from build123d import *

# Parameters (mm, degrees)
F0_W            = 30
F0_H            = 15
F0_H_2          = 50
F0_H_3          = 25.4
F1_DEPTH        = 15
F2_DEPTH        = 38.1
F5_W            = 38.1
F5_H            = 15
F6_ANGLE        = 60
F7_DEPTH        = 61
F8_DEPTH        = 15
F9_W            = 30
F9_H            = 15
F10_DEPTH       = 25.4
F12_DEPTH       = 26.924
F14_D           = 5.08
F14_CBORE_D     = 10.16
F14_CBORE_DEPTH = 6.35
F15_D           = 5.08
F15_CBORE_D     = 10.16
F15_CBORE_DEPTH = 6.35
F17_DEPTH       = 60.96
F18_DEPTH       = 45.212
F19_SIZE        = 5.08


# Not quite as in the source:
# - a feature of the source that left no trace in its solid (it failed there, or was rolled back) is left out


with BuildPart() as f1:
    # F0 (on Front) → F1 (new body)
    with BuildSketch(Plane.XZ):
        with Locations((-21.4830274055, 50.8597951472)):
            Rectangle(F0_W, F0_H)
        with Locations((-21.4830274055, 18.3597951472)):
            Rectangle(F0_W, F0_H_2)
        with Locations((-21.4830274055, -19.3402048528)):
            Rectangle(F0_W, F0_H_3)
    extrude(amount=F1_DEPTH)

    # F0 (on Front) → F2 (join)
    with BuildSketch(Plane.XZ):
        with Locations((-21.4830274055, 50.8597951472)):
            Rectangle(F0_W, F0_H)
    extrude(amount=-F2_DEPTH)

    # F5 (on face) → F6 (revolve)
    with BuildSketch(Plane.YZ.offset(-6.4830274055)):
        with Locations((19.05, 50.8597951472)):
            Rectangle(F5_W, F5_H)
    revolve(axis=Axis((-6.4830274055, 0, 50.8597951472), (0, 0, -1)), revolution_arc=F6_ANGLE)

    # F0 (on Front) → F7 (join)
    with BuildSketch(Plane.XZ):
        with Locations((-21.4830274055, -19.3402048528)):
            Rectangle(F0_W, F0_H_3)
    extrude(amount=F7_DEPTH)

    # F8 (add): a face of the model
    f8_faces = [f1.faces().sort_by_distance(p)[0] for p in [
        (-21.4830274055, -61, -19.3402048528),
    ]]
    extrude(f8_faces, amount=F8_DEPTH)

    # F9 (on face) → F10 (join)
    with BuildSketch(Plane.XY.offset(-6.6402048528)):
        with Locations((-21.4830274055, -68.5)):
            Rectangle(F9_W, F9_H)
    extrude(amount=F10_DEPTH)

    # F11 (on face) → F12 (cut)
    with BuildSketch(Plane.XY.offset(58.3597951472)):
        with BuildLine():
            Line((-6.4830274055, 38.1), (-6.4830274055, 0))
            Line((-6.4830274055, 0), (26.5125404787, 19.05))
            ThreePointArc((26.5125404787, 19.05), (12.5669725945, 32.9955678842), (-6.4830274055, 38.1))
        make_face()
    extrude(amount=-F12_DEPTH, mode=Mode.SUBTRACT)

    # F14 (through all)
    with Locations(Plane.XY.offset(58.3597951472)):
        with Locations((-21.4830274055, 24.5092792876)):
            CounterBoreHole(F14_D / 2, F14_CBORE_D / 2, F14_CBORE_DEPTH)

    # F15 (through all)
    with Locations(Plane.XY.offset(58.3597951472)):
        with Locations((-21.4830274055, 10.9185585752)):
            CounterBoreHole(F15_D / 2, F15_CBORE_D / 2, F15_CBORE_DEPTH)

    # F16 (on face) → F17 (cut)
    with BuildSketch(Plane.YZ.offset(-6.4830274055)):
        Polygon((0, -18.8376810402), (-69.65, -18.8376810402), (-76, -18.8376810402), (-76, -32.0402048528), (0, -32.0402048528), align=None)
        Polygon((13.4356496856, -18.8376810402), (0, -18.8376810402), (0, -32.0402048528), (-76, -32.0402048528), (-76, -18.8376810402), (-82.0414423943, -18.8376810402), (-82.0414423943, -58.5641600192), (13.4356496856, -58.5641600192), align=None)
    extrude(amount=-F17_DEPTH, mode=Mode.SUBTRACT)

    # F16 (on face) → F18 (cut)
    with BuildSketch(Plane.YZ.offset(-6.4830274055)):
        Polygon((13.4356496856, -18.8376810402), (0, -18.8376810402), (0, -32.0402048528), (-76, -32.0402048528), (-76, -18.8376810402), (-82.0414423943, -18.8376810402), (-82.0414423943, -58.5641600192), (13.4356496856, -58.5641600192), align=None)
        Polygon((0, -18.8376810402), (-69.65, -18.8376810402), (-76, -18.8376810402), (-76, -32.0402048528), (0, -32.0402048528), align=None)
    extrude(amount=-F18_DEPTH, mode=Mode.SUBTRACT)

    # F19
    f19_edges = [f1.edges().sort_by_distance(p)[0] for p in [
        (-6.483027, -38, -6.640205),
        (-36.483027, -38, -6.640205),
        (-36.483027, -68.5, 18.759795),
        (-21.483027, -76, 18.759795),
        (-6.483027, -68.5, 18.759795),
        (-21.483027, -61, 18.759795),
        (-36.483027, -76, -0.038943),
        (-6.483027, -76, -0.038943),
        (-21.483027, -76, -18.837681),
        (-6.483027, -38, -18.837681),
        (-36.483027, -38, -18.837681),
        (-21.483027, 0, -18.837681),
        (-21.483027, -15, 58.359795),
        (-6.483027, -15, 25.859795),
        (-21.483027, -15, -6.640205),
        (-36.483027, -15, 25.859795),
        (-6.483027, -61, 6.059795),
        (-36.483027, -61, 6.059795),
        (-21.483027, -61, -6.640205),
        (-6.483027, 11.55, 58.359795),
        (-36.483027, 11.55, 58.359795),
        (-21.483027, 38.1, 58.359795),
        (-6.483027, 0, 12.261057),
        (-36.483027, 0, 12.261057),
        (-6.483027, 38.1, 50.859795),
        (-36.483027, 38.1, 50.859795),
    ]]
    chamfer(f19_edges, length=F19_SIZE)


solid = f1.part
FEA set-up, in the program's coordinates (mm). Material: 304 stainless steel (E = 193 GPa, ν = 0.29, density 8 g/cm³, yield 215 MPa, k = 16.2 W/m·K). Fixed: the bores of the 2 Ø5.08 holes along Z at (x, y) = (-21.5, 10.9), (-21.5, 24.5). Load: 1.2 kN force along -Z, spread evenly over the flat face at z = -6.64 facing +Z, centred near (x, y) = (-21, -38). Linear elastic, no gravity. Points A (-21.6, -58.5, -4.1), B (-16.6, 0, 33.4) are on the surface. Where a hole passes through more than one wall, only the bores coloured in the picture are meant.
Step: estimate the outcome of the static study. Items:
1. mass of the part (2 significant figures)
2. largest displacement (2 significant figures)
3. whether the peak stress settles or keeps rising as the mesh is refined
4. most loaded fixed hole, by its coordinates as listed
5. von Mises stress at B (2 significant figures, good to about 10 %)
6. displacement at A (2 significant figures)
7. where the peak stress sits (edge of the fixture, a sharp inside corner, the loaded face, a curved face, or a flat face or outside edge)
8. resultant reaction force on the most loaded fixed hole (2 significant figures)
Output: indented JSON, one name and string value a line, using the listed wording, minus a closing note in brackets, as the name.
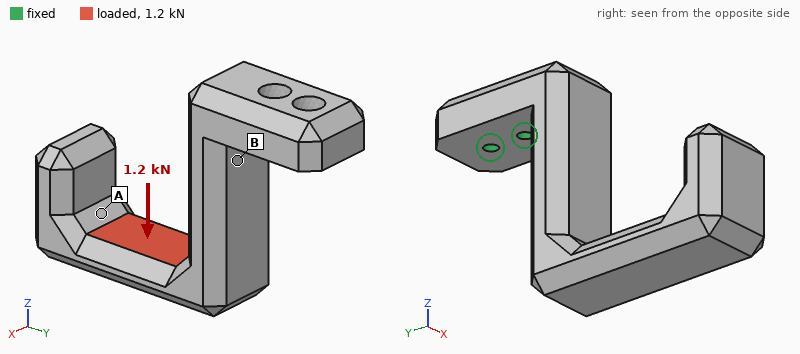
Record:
{
  "mass of the part": "590 g",
  "largest displacement": "0.25 mm",
  "whether the peak stress settles or keeps rising as the mesh is refined": "keeps rising",
  "most loaded fixed hole, by its coordinates as listed": "(-21.5, 10.9)",
  "von Mises stress at B": "38 MPa",
  "displacement at A": "0.19 mm",
  "where the peak stress sits": "edge of the fixture",
  "resultant reaction force on the most loaded fixed hole": "3.5 kN"
}
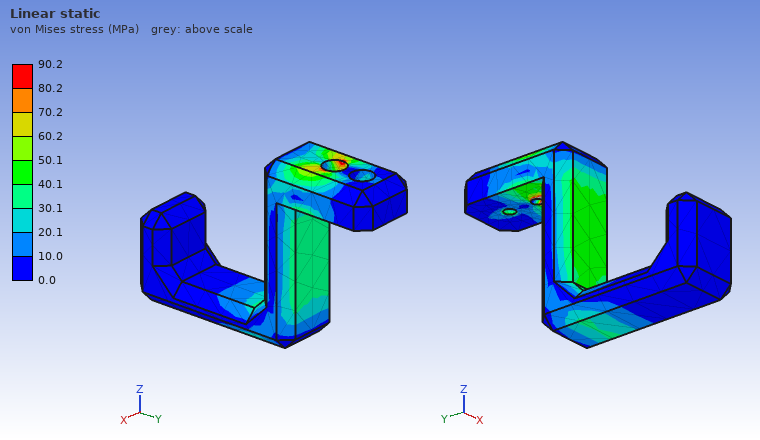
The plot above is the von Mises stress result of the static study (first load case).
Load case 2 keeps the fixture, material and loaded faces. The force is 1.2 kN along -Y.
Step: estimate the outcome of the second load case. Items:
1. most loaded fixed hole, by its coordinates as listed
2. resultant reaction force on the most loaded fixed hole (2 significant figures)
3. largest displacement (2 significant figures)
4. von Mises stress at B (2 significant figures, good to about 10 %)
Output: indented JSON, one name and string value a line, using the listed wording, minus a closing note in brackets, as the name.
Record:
{
  "most loaded fixed hole, by its coordinates as listed": "(-21.5, 10.9)",
  "resultant reaction force on the most loaded fixed hole": "3.4 kN",
  "largest displacement": "0.23 mm",
  "von Mises stress at B": "53 MPa"
}
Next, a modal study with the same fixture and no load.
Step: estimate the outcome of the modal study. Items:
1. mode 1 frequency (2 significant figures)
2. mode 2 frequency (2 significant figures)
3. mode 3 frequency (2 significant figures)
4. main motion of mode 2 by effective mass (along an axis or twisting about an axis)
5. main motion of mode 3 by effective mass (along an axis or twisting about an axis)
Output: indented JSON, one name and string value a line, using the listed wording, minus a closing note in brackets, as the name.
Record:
{
  "mode 1 frequency": "580 Hz",
  "mode 2 frequency": "760 Hz",
  "mode 3 frequency": "1500 Hz",
  "main motion of mode 2 by effective mass": "along X",
  "main motion of mode 3 by effective mass": "along Y"
}
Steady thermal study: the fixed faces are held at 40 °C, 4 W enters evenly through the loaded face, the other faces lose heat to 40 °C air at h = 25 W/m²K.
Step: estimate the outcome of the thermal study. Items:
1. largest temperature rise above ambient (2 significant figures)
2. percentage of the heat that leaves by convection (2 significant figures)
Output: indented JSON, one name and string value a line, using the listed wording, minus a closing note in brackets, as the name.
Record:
{
  "largest temperature rise above ambient": "20 K",
  "percentage of the heat that leaves by convection": "81 %"
}
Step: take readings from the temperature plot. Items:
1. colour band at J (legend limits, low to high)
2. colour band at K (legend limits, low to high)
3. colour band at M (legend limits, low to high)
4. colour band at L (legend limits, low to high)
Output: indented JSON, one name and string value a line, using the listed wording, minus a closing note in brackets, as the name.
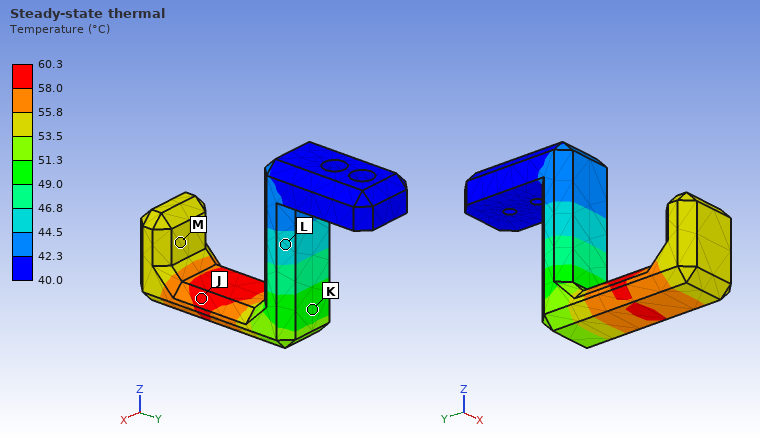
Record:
{
  "colour band at J": "58.0 to 60.3 °C",
  "colour band at K": "49.0 to 51.3 °C",
  "colour band at M": "53.5 to 55.8 °C",
  "colour band at L": "44.5 to 46.8 °C"
}
